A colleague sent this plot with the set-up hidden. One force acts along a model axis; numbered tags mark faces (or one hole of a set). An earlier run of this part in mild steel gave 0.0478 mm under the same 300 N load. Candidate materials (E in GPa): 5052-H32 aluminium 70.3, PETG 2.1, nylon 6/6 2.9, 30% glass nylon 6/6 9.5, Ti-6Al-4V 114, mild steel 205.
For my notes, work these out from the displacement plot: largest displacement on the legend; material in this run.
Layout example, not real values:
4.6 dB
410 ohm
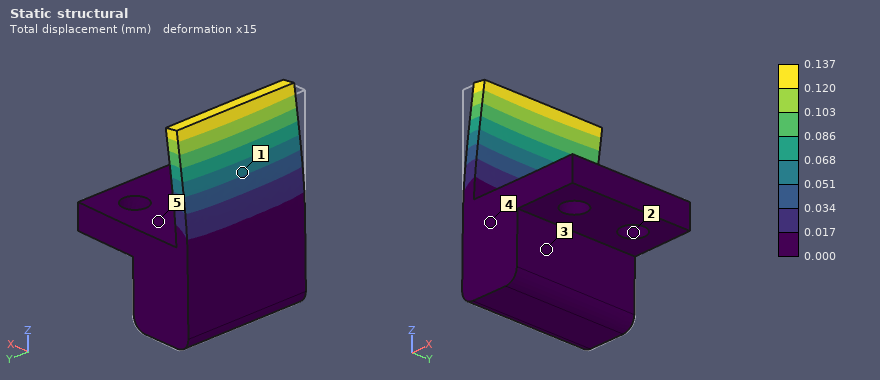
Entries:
0.137 mm
5052-H32 aluminium
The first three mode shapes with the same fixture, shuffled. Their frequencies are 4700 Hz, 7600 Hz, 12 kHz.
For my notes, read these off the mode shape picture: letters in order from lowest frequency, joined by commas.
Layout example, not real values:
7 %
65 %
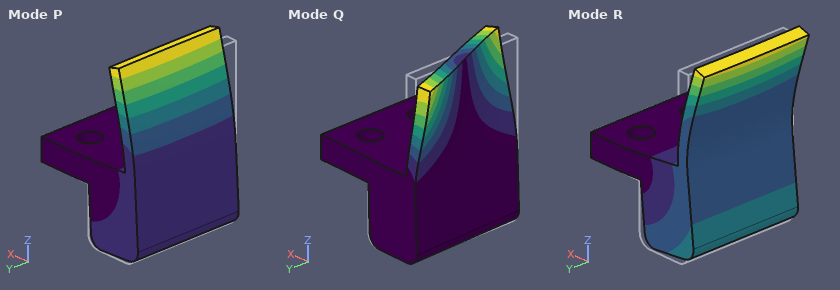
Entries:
P, R, Q
